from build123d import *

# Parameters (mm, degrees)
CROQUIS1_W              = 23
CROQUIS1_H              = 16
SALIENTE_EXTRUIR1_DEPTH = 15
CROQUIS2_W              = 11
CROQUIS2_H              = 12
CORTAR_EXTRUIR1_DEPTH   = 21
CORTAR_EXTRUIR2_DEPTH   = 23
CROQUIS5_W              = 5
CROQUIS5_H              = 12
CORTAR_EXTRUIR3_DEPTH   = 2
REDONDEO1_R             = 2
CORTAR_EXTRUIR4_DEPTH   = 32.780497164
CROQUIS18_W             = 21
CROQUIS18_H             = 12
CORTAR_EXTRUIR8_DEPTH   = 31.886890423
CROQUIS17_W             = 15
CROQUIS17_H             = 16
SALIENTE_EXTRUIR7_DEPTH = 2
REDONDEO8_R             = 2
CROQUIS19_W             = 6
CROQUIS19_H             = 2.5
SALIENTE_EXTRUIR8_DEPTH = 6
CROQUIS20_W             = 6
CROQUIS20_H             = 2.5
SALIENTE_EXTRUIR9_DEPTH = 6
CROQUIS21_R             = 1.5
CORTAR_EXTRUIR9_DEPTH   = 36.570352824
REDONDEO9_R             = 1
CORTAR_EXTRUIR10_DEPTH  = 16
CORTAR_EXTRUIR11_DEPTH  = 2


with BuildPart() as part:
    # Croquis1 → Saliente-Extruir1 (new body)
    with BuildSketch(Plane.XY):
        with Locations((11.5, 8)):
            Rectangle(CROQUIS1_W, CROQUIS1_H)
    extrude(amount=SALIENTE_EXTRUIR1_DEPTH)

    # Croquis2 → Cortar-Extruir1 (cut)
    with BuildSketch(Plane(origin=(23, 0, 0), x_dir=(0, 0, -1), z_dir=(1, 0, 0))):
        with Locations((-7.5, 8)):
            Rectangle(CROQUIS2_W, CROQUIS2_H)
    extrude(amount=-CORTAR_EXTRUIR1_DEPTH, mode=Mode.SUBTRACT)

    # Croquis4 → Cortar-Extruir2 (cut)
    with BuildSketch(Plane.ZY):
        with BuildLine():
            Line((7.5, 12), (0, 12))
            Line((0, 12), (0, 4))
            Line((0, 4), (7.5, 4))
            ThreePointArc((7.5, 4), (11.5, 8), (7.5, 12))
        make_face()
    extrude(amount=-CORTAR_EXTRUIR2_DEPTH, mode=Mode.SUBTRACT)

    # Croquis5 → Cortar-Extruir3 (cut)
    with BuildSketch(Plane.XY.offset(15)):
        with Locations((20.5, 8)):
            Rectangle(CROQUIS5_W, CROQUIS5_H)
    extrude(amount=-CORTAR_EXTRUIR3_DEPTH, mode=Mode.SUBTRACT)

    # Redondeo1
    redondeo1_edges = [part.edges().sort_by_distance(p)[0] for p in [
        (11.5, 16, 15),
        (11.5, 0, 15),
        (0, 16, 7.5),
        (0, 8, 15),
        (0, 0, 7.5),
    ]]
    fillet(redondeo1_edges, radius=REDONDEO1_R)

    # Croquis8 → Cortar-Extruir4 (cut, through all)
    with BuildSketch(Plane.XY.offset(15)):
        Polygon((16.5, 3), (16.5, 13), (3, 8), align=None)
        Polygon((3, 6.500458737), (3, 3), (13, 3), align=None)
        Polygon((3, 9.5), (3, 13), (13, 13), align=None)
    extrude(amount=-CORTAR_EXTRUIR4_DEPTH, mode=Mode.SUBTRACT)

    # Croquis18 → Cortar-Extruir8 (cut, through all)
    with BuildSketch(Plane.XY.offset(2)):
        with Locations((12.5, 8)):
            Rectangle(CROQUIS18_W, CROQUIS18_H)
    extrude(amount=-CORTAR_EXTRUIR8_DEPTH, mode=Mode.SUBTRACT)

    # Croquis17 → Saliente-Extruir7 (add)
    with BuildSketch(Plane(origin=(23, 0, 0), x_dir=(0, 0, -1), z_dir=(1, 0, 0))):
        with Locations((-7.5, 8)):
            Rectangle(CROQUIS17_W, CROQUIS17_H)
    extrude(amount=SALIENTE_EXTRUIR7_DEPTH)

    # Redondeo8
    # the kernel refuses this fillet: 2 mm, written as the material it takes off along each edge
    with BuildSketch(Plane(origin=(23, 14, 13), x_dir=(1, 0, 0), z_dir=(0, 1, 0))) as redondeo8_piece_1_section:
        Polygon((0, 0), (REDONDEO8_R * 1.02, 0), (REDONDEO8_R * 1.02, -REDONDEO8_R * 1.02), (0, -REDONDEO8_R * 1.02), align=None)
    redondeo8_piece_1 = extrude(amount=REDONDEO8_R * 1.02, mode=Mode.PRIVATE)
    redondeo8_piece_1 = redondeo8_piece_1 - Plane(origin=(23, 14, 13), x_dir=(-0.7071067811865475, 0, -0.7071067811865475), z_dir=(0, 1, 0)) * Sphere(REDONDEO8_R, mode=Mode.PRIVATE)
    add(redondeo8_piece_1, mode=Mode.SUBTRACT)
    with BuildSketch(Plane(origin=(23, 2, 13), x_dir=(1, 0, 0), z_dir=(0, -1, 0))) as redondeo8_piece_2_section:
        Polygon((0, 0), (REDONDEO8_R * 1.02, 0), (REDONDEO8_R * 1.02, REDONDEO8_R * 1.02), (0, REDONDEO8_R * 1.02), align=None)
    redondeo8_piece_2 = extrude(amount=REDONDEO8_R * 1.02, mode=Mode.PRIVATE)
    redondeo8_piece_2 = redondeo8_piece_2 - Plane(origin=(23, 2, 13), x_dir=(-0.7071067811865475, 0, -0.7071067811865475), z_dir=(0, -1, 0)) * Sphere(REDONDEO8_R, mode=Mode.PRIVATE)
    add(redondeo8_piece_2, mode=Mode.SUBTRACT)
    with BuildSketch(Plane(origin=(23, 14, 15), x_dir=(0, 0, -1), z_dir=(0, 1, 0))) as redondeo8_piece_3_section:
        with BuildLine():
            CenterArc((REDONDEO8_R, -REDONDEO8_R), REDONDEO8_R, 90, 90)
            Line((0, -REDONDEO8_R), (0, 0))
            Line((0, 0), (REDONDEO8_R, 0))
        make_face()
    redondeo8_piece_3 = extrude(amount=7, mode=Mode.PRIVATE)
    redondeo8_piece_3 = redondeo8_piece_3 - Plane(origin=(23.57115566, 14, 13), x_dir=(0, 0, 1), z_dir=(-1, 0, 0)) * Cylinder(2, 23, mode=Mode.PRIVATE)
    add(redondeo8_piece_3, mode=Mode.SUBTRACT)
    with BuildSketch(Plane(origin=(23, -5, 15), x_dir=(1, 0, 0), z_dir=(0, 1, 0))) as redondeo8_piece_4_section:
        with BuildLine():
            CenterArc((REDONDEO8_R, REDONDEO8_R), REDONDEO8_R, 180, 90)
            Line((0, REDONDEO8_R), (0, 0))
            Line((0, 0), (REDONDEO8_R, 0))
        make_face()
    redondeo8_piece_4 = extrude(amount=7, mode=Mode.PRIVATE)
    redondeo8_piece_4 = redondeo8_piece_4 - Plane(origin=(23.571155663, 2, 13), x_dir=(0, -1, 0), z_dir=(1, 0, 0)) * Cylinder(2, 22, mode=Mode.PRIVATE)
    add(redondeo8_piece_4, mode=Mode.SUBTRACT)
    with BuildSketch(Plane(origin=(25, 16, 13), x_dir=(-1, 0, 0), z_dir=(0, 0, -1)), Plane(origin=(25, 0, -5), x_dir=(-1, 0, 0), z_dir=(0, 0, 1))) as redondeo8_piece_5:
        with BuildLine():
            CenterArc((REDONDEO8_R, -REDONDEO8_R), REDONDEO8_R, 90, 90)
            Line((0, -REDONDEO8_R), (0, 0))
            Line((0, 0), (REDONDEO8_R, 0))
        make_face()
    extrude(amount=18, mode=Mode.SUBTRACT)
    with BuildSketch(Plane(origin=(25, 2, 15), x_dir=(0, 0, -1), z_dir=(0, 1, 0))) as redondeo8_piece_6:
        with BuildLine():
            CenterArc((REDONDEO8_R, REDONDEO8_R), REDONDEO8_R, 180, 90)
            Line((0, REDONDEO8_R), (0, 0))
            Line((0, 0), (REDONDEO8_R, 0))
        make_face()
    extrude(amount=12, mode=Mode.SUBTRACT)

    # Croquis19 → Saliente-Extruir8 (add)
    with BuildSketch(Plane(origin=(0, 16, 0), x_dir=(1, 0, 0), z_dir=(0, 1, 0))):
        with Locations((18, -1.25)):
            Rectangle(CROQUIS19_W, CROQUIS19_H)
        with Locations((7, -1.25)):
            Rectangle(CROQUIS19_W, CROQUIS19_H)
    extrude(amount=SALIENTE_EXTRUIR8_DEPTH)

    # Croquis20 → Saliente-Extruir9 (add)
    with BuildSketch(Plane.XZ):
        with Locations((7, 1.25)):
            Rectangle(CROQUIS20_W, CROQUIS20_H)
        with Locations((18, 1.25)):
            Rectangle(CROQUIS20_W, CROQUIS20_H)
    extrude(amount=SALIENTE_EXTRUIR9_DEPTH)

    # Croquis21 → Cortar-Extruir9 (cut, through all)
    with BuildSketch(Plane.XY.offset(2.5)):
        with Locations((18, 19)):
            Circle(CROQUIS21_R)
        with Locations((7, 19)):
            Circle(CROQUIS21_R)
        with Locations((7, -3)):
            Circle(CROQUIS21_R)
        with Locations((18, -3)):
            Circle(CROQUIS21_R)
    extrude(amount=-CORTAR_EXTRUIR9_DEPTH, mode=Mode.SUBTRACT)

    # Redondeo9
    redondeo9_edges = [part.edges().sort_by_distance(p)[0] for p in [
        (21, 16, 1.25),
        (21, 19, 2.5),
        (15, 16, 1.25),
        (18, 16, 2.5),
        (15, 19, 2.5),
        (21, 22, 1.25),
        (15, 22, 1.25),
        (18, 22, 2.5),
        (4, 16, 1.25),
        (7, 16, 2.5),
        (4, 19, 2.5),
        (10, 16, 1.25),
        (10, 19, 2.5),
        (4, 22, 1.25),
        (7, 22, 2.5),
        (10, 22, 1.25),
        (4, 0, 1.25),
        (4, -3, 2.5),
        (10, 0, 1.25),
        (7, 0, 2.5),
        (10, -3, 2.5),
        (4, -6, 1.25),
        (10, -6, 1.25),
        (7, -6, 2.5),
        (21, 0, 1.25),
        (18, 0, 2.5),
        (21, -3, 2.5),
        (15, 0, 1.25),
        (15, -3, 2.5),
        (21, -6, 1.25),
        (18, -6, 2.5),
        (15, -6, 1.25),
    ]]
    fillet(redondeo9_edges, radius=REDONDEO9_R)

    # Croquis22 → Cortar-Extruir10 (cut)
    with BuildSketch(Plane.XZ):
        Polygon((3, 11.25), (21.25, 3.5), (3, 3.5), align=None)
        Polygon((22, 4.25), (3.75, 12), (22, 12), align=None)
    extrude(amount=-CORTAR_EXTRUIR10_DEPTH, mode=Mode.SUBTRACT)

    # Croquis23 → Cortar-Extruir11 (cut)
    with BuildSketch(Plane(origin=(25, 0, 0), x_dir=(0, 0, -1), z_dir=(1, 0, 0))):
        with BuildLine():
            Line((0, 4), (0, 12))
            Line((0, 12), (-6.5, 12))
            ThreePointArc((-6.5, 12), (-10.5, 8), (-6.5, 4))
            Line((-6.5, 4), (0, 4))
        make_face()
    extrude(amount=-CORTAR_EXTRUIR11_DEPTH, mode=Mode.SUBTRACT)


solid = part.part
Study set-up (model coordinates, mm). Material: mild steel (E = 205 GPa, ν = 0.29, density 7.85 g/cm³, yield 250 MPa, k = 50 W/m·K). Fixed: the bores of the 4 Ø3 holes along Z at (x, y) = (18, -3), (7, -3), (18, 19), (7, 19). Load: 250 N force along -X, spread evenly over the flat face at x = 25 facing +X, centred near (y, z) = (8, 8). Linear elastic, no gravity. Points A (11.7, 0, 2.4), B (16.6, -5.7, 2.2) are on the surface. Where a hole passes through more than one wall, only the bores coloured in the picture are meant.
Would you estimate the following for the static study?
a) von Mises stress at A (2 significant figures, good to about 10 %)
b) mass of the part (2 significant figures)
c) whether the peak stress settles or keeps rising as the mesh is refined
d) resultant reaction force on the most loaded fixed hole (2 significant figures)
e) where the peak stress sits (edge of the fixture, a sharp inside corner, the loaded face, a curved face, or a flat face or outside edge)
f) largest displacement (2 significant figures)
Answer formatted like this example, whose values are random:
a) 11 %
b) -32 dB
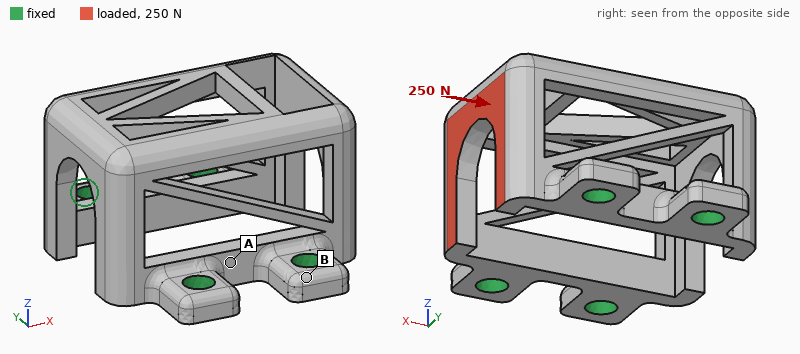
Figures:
a) 13 MPa
b) 13 g
c) keeps rising
d) 93 N
e) a sharp inside corner
f) 13 µm
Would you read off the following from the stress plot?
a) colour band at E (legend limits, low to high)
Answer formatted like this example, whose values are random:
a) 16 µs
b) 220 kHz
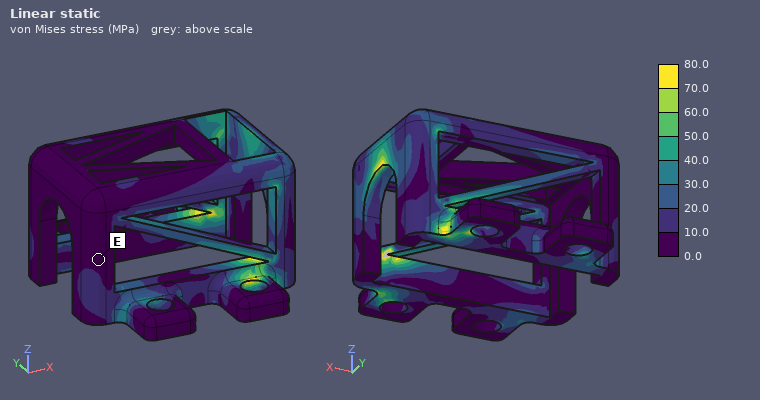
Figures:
a) 0.0 to 10.0 MPa
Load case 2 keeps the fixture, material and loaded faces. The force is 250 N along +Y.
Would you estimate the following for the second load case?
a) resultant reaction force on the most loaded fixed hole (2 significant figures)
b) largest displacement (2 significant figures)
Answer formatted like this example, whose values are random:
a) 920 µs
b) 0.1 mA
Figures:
a) 170 N
b) 11 µm
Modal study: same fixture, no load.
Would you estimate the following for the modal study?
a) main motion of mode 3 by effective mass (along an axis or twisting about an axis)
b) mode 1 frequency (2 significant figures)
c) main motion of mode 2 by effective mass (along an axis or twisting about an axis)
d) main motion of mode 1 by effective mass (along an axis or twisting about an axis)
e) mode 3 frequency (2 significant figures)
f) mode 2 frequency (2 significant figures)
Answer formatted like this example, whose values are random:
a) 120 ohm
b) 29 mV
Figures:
a) along Z
b) 8500 Hz
c) along Y
d) along X
e) 12 kHz
f) 9500 Hz
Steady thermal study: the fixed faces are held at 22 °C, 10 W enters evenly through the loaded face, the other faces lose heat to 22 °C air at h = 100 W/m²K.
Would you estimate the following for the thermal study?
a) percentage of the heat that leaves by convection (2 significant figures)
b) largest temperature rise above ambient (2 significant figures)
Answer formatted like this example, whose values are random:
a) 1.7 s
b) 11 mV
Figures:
a) 43 %
b) 69 K
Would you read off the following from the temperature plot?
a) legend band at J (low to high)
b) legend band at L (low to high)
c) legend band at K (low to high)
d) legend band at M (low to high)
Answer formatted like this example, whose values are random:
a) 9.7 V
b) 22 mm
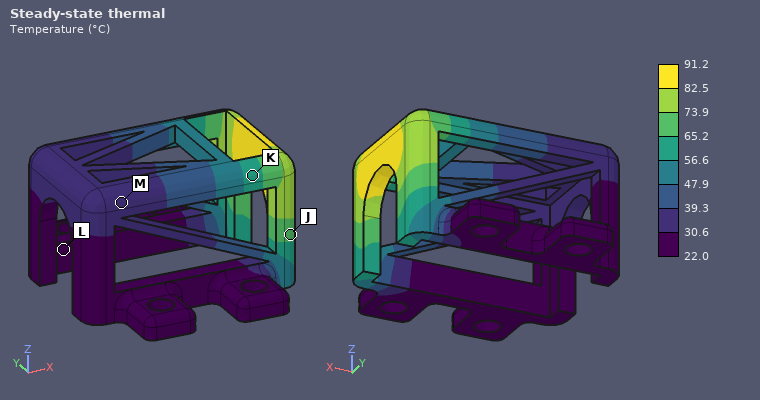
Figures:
a) 65.2 to 73.9 °C
b) 22.0 to 30.6 °C
c) 56.6 to 65.2 °C
d) 30.6 to 39.3 °C
